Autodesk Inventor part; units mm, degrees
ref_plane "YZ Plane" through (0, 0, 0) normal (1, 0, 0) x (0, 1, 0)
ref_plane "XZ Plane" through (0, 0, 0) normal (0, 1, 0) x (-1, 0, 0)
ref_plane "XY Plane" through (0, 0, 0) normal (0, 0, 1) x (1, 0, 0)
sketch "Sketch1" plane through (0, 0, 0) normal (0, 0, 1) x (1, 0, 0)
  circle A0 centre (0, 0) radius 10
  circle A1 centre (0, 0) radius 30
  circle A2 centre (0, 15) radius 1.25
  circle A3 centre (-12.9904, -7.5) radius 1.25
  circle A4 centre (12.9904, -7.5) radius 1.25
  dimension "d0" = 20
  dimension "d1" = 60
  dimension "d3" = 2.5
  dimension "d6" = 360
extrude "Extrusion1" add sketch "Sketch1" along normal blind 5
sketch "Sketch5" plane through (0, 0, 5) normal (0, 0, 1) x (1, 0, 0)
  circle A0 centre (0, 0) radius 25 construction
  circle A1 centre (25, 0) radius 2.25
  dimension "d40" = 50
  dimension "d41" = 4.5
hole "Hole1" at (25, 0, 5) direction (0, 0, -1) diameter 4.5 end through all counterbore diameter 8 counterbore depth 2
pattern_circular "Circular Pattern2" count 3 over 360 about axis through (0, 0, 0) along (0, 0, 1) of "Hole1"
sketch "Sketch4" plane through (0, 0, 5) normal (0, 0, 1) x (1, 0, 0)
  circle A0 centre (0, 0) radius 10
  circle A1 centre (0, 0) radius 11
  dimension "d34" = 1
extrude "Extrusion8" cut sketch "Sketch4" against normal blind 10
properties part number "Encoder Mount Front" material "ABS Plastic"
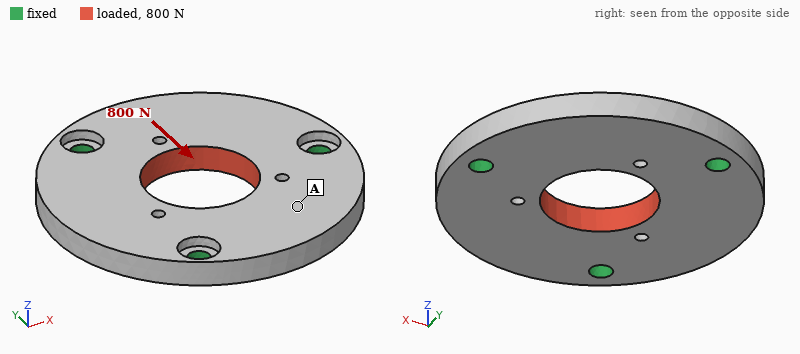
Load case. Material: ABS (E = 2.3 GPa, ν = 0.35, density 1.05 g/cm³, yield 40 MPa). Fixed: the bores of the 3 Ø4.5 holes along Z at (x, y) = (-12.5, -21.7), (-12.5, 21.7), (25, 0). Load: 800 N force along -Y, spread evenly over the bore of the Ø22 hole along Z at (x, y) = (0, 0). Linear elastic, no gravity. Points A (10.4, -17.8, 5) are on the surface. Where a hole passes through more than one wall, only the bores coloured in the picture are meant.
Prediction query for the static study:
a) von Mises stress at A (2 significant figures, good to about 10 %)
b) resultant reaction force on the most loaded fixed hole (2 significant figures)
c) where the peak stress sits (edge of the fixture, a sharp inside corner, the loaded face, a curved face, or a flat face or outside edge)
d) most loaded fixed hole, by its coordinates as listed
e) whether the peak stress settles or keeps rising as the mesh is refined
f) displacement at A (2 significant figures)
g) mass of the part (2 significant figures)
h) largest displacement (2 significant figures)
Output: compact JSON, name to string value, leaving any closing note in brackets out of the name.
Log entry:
{"von Mises stress at A": "1.8 MPa", "resultant reaction force on the most loaded fixed hole": "290 N", "where the peak stress sits": "edge of the fixture", "most loaded fixed hole, by its coordinates as listed": "(25, 0)", "whether the peak stress settles or keeps rising as the mesh is refined": "keeps rising", "displacement at A": "56 µm", "mass of the part": "12 g", "largest displacement": "65 µm"}
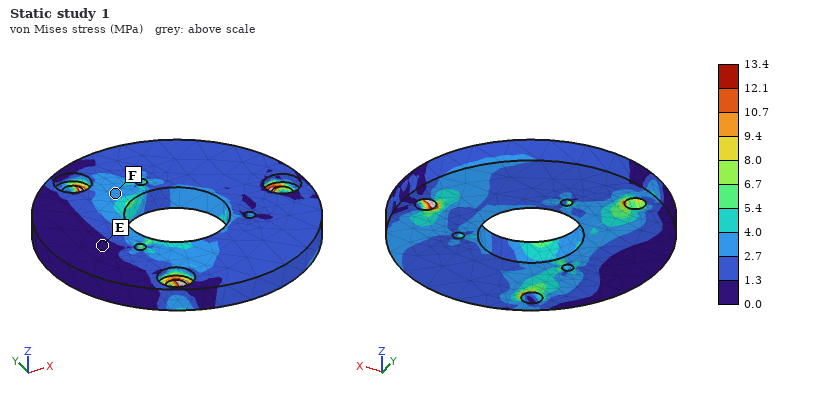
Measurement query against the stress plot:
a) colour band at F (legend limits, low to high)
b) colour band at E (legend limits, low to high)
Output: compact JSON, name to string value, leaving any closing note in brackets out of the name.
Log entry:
{"colour band at F": "2.7 to 4.0 MPa", "colour band at E": "0.0 to 1.3 MPa"}
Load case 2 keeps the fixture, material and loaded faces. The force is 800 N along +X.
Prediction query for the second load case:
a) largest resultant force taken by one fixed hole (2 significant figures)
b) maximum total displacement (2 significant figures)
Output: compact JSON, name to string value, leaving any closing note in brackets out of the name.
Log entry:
{"largest resultant force taken by one fixed hole": "280 N", "maximum total displacement": "74 µm"}
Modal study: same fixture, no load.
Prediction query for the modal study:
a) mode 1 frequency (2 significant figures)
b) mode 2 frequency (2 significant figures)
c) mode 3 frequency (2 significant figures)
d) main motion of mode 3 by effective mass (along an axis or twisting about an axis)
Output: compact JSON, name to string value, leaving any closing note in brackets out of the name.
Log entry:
{"mode 1 frequency": "2100 Hz", "mode 2 frequency": "2100 Hz", "mode 3 frequency": "2600 Hz", "main motion of mode 3 by effective mass": "along Z"}
